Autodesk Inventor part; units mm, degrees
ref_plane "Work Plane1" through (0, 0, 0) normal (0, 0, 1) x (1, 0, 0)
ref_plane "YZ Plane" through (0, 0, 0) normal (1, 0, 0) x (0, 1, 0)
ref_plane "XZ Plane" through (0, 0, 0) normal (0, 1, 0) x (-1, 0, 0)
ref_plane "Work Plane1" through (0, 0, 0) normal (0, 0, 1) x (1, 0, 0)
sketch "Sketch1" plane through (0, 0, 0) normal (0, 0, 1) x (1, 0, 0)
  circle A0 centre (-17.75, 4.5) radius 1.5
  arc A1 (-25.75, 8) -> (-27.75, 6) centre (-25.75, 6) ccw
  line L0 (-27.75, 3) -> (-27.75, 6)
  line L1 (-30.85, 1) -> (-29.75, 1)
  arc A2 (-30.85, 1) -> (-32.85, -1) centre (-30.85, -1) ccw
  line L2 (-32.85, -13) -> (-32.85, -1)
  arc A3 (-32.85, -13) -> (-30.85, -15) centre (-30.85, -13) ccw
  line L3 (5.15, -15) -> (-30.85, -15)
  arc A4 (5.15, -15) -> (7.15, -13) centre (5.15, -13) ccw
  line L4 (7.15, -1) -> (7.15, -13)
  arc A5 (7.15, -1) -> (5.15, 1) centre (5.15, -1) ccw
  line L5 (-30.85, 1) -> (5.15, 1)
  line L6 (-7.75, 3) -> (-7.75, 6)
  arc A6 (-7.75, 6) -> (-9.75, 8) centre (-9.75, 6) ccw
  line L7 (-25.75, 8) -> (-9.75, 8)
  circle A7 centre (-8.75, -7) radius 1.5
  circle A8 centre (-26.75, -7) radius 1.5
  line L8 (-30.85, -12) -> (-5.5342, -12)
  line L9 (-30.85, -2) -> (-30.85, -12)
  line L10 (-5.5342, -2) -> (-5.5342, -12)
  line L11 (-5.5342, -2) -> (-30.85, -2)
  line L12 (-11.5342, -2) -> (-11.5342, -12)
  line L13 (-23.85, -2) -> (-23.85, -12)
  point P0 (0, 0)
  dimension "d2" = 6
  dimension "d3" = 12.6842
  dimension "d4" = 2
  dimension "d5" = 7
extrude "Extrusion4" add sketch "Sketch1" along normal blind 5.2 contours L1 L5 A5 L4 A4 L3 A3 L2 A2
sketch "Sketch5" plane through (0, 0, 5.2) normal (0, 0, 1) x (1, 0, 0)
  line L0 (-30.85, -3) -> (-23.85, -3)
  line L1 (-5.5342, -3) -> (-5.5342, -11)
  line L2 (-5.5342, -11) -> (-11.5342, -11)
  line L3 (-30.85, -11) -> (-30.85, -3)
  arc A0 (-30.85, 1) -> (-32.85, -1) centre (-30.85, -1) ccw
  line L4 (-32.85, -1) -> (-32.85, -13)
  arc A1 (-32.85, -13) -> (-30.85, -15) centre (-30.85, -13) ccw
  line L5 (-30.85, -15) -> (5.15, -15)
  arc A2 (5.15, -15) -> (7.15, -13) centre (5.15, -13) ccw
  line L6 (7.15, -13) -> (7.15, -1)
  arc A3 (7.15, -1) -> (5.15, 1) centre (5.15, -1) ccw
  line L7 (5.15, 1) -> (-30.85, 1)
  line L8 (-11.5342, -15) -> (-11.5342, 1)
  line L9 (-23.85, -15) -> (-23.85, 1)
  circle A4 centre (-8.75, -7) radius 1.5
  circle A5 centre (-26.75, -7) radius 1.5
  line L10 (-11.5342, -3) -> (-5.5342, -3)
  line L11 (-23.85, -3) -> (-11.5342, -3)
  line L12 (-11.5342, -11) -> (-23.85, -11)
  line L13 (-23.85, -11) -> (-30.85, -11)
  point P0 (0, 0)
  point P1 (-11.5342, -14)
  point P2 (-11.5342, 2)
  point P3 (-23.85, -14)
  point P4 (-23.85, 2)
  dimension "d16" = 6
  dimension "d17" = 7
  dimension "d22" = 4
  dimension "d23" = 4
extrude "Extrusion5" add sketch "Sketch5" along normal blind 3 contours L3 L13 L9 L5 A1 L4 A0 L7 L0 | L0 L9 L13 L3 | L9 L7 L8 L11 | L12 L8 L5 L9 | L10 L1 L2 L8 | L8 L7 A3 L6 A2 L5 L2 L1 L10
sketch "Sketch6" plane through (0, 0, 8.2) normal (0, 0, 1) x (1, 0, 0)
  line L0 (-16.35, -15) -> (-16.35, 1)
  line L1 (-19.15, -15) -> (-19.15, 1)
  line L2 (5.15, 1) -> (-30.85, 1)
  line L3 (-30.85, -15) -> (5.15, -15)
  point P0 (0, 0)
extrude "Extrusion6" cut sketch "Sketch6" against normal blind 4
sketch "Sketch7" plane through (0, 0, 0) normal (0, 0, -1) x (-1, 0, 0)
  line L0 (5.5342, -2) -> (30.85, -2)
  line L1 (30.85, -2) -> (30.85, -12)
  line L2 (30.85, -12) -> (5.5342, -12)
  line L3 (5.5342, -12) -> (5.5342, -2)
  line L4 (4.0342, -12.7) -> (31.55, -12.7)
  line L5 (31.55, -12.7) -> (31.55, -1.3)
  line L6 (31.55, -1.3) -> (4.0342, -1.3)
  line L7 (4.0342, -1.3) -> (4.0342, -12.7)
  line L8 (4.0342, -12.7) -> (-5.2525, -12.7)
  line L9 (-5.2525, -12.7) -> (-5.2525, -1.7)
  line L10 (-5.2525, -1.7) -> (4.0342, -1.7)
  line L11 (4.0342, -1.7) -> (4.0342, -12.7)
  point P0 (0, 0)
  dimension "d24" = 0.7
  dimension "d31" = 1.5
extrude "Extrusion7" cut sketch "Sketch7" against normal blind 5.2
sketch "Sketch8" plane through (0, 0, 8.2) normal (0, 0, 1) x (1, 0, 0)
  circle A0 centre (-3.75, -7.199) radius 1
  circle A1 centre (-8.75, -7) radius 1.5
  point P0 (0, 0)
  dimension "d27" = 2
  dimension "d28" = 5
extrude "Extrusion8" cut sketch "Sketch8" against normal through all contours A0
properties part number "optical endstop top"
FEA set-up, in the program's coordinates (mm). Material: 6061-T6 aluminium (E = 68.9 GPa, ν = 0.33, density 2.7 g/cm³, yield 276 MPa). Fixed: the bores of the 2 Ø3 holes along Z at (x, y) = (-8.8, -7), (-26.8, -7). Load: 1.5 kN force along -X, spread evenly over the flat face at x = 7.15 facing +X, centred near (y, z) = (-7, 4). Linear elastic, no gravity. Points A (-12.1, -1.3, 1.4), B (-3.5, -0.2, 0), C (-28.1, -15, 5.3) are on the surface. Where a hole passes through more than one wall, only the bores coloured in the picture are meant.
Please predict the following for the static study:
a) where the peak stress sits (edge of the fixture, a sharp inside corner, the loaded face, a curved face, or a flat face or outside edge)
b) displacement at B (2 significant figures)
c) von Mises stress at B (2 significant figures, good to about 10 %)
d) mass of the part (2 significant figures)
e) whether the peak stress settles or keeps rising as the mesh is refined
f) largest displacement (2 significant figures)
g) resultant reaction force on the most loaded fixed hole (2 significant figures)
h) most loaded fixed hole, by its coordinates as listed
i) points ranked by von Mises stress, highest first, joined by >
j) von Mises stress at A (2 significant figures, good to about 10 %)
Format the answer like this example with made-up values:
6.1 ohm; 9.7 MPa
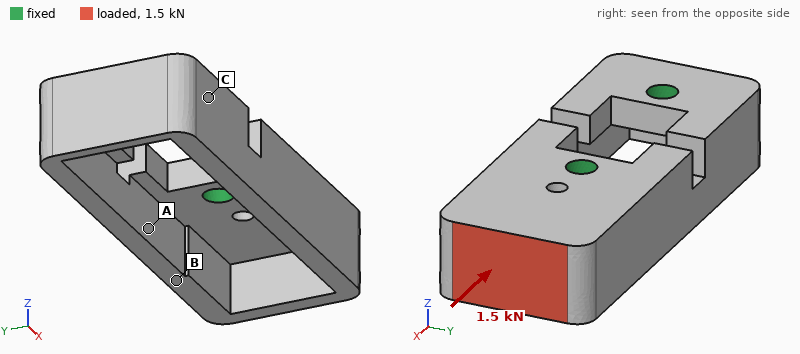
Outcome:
edge of the fixture; 17 µm; 54 MPa; 7.1 g; keeps rising; 64 µm; 1.1 kN; (-8.8, -7); B > A > C; 25 MPa
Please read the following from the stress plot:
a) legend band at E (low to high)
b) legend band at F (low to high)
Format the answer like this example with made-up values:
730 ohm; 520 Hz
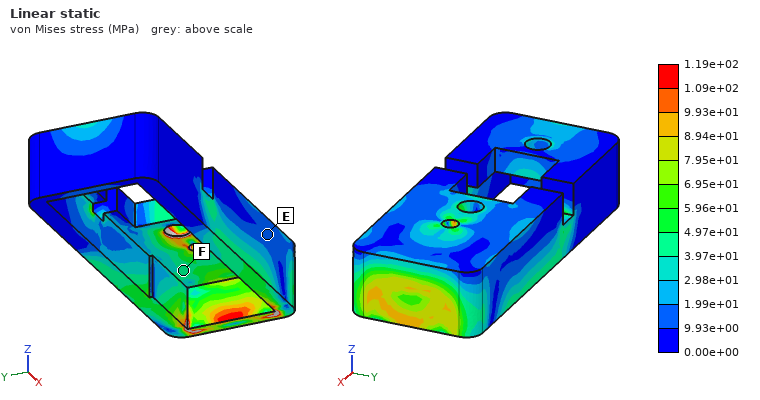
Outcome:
9.93e+00 to 1.99e+01 MPa; 3.97e+01 to 4.97e+01 MPa
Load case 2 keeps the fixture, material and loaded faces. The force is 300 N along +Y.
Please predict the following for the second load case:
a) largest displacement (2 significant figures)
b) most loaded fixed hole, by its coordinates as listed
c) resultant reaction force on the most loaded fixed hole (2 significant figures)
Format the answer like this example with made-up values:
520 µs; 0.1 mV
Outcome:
52 µm; (-8.8, -7); 360 N
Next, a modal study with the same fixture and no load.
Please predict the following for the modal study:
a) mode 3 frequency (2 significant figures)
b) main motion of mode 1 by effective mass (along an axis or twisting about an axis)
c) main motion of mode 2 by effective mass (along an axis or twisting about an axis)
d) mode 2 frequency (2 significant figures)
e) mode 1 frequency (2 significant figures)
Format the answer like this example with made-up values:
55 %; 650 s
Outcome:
14 kHz; along Y; along Z; 11 kHz; 9900 Hz
